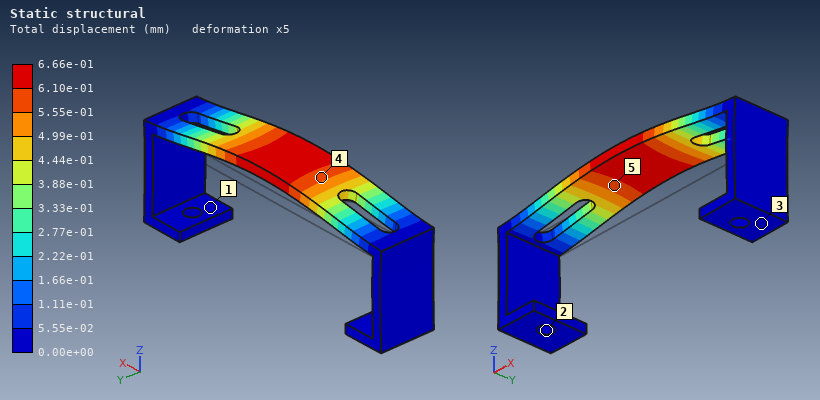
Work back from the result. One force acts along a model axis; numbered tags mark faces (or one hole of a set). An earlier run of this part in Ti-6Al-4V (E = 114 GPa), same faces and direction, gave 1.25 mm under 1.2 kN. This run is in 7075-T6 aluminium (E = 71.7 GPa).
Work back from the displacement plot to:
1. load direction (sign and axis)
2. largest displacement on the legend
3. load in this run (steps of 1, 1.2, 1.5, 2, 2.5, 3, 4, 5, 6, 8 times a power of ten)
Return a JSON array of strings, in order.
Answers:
["+Z", "6.66e-01 mm", "400 N"]
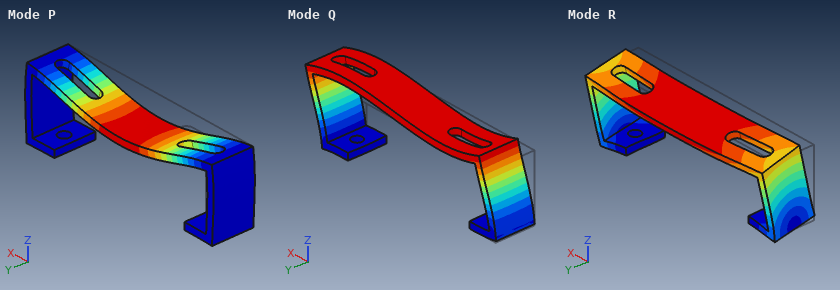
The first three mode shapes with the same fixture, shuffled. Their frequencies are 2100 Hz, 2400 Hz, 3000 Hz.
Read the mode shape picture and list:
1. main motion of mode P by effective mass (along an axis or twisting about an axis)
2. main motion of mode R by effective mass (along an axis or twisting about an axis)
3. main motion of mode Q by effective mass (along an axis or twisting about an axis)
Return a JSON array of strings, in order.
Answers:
["along Z", "along Y", "along X"]
